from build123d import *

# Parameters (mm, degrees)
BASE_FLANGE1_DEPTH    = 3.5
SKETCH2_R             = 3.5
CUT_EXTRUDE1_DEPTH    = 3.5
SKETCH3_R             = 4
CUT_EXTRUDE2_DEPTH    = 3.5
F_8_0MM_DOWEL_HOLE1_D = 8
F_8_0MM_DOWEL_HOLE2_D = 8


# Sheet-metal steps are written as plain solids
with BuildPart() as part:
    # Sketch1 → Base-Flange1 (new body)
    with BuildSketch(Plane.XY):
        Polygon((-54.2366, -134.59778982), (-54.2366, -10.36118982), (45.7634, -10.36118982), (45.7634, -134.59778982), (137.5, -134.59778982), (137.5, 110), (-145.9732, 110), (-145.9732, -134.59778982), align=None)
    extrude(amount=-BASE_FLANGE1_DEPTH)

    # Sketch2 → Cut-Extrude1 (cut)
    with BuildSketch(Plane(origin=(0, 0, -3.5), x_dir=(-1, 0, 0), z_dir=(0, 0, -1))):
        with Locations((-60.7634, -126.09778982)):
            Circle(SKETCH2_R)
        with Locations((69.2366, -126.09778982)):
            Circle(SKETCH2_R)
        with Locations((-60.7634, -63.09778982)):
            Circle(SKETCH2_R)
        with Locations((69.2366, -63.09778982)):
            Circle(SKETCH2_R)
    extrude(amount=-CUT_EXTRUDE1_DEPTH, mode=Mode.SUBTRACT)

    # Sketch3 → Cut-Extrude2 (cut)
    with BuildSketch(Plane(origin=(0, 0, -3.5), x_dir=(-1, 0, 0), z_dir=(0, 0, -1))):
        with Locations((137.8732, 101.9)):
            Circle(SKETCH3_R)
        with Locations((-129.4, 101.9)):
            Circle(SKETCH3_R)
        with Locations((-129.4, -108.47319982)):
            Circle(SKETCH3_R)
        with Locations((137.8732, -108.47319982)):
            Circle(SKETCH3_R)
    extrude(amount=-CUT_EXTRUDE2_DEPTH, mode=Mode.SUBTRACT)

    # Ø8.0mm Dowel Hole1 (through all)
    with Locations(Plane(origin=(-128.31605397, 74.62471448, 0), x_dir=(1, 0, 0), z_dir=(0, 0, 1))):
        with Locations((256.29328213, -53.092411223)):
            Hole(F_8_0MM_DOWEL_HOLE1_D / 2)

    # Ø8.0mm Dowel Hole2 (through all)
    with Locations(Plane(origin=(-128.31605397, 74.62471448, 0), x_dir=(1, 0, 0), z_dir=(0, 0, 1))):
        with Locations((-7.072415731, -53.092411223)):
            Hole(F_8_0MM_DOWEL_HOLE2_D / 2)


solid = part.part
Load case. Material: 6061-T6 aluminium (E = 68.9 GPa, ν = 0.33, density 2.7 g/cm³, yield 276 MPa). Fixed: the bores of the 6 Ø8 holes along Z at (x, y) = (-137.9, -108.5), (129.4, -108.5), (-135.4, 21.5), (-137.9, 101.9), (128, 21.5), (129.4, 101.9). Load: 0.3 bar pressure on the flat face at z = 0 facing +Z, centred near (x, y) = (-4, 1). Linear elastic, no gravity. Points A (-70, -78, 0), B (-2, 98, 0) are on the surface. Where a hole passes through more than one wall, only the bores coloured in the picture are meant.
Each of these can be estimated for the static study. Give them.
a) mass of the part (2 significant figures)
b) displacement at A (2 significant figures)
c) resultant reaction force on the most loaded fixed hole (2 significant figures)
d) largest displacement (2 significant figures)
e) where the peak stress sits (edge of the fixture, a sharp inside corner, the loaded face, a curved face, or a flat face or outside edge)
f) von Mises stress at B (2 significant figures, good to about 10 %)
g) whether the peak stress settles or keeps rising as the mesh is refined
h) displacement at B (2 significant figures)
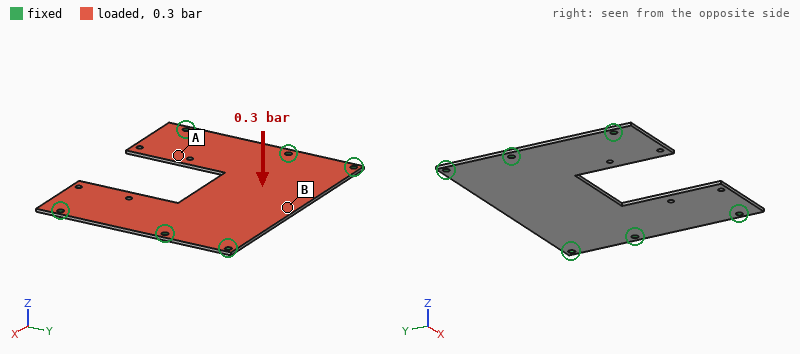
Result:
530 g
1.0 mm
430 N
1.9 mm
edge of the fixture
45 MPa
keeps rising
1.7 mm
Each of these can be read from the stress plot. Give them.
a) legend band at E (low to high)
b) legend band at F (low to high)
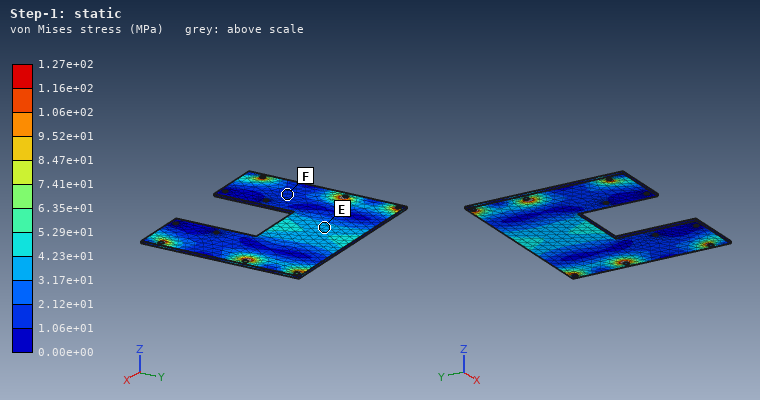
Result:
3.17e+01 to 4.23e+01 MPa
1.06e+01 to 2.12e+01 MPa
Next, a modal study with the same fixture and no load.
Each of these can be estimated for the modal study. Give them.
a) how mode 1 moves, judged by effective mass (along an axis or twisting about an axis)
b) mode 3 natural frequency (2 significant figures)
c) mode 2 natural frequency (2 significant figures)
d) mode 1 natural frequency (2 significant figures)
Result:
along Z
450 Hz
390 Hz
260 Hz
